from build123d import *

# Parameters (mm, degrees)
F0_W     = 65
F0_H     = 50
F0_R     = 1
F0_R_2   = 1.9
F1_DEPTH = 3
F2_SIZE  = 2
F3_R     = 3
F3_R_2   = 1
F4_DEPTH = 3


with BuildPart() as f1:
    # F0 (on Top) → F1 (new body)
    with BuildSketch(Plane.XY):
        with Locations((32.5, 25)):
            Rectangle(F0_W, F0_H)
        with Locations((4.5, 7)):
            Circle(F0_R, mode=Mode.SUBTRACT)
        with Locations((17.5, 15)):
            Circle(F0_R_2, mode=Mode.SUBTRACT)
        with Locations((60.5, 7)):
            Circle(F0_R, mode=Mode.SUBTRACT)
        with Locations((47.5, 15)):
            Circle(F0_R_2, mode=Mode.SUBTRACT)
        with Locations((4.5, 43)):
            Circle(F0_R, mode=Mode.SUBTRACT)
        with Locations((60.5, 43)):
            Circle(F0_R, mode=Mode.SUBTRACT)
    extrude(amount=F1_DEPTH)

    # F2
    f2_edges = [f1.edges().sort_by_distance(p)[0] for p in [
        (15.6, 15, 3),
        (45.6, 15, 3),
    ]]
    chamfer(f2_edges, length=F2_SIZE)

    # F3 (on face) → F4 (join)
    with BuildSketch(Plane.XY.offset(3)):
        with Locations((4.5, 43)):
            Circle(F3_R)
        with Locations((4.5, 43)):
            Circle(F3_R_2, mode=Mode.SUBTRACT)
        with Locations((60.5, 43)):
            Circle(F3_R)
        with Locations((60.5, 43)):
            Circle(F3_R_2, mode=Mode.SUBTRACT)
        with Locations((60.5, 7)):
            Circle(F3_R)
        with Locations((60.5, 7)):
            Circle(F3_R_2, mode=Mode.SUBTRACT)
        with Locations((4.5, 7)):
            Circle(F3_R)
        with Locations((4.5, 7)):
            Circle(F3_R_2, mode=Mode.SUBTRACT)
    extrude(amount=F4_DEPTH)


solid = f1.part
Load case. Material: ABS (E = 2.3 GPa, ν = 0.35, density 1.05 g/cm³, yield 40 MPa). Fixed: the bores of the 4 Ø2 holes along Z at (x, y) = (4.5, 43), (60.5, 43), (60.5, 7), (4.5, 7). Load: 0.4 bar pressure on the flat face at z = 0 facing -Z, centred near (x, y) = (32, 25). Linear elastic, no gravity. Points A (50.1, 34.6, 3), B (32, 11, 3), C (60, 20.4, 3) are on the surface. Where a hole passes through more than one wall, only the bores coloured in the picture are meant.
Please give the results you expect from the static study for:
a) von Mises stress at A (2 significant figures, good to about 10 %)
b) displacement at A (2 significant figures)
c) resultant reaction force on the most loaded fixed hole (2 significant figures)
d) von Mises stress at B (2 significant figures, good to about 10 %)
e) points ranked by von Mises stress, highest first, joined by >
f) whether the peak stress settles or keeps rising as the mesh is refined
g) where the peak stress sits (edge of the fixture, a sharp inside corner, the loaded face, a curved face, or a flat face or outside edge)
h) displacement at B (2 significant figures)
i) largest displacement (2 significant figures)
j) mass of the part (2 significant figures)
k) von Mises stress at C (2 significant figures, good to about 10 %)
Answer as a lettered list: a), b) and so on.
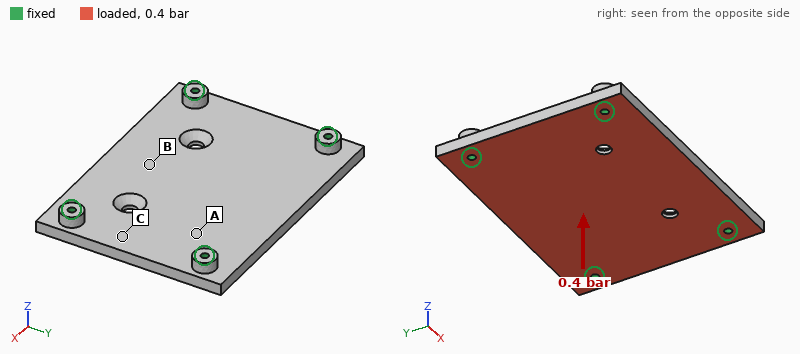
a) 0.88 MPa
b) 0.12 mm
c) 34 N
d) 3.4 MPa
e) B > C > A
f) keeps rising
g) edge of the fixture
h) 0.24 mm
i) 0.26 mm
j) 10 g
k) 1.7 MPa
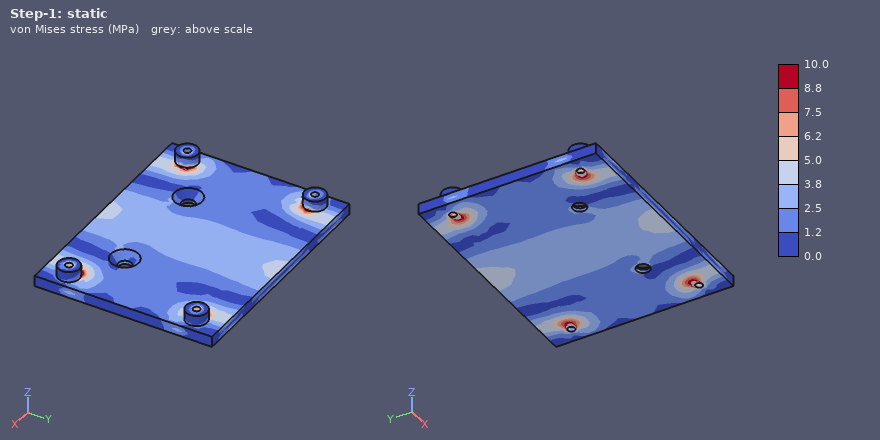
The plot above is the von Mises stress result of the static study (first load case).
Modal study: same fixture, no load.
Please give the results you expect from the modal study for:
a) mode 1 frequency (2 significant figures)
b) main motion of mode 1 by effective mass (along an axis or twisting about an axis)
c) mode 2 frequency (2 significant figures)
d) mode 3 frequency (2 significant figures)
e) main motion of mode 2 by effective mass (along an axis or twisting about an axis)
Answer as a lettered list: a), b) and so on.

a) 1300 Hz
b) along Z
c) 1800 Hz
d) 2700 Hz
e) twisting about X
